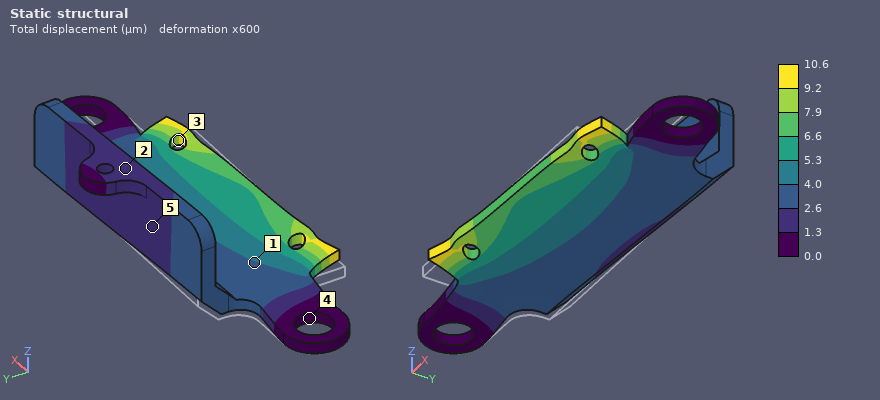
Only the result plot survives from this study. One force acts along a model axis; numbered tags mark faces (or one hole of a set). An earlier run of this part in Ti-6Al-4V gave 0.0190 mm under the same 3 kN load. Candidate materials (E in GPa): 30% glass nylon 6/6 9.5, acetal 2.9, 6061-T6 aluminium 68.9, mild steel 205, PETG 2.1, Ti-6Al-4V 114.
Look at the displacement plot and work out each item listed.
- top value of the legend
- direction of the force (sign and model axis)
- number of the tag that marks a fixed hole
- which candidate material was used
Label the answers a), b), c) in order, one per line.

a) 10.6 µm
b) +X
c) 4
d) mild steel
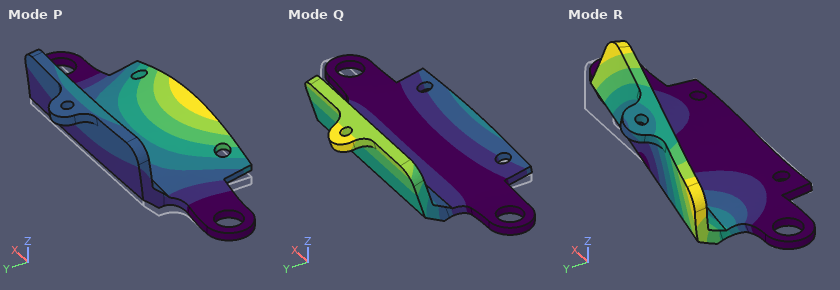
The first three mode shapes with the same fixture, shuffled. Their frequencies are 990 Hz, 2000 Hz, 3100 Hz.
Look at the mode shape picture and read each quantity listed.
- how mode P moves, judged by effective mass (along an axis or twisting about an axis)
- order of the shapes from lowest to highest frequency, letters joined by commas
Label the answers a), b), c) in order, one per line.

a) along Z
b) Q, P, R
